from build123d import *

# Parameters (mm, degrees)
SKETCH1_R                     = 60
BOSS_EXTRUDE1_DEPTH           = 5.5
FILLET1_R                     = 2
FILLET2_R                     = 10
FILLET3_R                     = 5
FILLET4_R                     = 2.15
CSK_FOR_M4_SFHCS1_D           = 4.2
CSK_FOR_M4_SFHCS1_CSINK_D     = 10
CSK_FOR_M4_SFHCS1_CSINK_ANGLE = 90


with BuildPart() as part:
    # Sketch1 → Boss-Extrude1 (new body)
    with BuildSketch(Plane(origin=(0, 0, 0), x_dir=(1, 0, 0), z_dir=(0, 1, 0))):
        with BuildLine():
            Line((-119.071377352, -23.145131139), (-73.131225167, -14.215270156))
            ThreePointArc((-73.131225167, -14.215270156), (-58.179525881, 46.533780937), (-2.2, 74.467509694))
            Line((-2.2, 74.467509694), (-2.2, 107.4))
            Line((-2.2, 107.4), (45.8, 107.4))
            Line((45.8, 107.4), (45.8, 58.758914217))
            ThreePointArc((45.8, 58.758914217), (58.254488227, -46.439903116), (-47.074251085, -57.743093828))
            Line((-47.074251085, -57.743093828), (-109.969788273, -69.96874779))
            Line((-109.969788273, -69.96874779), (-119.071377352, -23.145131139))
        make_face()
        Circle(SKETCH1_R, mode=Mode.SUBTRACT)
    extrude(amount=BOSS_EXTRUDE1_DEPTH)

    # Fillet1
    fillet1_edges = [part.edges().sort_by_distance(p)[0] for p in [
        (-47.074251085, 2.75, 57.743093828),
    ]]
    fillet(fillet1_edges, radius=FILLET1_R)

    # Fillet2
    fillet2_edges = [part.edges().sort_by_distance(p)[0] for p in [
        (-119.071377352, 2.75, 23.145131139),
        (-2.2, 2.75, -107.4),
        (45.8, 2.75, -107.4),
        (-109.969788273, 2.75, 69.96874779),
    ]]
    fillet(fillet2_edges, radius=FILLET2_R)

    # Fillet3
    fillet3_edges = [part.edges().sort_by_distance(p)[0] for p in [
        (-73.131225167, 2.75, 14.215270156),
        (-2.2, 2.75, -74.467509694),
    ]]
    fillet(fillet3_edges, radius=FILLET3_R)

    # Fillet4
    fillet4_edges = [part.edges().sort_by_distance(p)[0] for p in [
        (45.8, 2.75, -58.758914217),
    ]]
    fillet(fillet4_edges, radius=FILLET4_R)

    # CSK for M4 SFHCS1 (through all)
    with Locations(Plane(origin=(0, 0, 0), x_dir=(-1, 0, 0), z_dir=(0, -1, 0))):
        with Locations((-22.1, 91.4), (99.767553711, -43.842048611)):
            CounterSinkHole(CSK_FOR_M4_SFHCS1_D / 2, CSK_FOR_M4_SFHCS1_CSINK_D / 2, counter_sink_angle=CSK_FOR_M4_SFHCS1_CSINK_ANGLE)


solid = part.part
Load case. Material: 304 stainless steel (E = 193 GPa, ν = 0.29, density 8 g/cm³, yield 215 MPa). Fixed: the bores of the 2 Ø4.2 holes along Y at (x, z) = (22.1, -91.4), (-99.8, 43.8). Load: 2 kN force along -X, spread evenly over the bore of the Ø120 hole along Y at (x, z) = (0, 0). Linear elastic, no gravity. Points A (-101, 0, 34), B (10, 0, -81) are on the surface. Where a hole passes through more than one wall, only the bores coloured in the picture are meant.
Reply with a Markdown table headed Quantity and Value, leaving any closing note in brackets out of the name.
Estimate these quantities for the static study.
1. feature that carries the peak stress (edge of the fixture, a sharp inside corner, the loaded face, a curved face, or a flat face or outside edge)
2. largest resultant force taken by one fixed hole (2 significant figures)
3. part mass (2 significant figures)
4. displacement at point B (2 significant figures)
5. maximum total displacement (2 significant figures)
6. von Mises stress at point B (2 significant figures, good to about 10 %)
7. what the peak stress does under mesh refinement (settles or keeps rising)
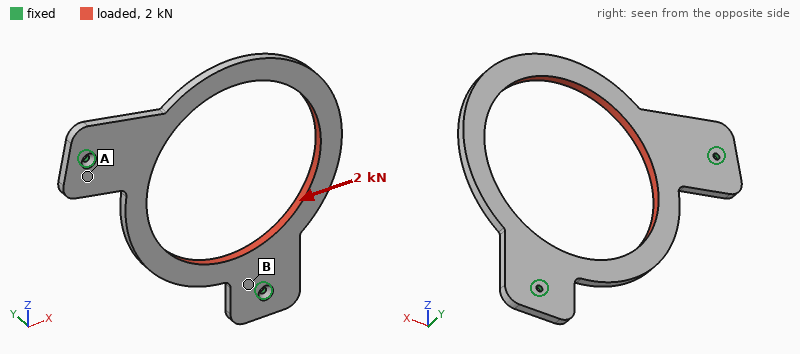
| Quantity | Value |
|---|---|
| feature that carries the peak stress | edge of the fixture |
| largest resultant force taken by one fixed hole | 1.1 kN |
| part mass | 450 g |
| displacement at point B | 10 µm |
| maximum total displacement | 48 µm |
| von Mises stress at point B | 12 MPa |
| what the peak stress does under mesh refinement | keeps rising |
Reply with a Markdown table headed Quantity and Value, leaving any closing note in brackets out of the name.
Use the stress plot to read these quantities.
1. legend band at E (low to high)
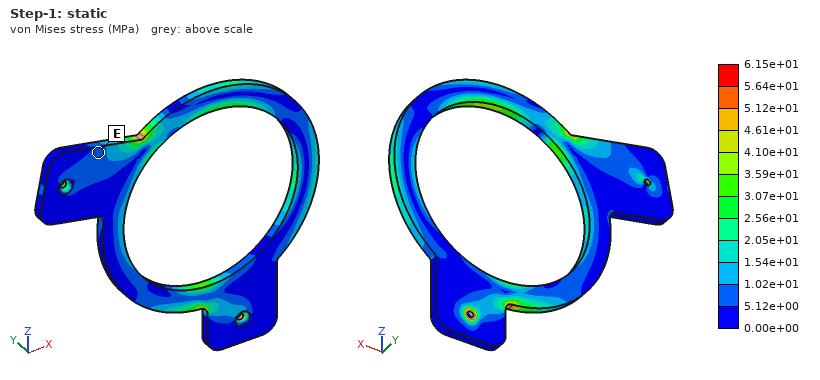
| Quantity | Value |
|---|---|
| legend band at E | 5.12e+00 to 1.02e+01 MPa |
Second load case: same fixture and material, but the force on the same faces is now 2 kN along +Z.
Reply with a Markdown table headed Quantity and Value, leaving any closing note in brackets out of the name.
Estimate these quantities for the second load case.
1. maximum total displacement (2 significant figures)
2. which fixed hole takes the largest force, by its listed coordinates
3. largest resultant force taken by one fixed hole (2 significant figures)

| Quantity | Value |
|---|---|
| maximum total displacement | 74 µm |
| which fixed hole takes the largest force, by its listed coordinates | (22.1, -91.4) |
| largest resultant force taken by one fixed hole | 1.3 kN |
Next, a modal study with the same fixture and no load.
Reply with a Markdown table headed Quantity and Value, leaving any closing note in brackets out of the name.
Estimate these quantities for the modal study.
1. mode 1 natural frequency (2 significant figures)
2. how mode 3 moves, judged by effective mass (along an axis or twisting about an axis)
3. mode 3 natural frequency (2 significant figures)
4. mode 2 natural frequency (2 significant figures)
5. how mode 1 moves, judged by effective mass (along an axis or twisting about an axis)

| Quantity | Value |
|---|---|
| mode 1 natural frequency | 250 Hz |
| how mode 3 moves, judged by effective mass | along Y |
| mode 3 natural frequency | 780 Hz |
| mode 2 natural frequency | 690 Hz |
| how mode 1 moves, judged by effective mass | along Y |
